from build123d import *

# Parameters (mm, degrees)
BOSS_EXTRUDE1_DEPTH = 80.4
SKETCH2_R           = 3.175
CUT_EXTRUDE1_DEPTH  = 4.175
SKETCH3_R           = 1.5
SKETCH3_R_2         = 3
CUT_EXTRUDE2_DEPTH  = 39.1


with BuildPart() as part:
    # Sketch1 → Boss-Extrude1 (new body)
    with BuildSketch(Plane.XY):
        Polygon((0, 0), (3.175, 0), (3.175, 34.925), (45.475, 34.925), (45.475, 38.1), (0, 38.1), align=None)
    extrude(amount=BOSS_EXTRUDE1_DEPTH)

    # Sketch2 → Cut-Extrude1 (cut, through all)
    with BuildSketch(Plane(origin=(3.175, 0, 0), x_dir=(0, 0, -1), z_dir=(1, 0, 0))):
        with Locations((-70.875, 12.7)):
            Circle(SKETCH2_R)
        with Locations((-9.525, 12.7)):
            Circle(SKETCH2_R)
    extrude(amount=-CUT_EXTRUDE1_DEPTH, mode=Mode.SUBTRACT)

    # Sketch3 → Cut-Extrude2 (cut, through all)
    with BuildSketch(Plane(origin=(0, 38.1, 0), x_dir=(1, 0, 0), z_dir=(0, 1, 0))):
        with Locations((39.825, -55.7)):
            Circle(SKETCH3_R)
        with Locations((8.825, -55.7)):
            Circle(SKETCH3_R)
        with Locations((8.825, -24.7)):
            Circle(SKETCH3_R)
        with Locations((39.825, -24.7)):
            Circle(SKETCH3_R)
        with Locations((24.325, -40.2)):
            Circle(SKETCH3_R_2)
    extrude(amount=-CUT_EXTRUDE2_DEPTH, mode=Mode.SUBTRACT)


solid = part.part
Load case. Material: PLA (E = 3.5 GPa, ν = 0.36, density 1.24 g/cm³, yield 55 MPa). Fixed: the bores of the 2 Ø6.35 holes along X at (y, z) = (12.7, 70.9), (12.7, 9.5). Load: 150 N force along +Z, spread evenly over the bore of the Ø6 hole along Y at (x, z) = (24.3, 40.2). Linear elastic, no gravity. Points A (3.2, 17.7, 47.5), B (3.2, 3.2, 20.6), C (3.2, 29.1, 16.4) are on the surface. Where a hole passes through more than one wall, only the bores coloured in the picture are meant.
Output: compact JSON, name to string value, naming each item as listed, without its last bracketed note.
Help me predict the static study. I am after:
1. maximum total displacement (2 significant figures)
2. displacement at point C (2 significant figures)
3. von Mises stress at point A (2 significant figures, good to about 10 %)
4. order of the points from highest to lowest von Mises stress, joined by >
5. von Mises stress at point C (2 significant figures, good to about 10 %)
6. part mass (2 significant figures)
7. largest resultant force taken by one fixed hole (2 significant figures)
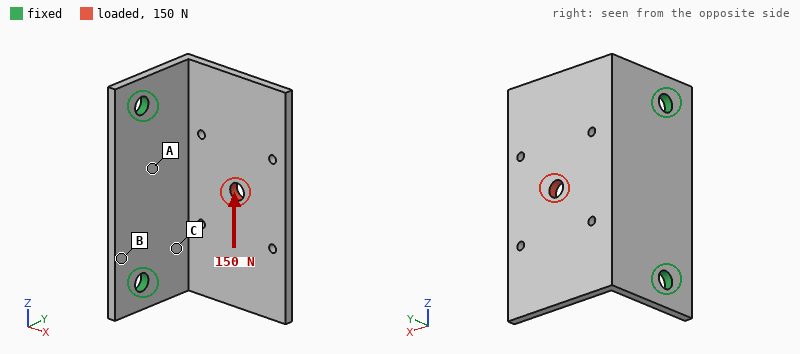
{"maximum total displacement": "1.0 mm", "displacement at point C": "0.20 mm", "von Mises stress at point A": "4.0 MPa", "order of the points from highest to lowest von Mises stress, joined by >": "C > A > B", "von Mises stress at point C": "7.6 MPa", "part mass": "25 g", "largest resultant force taken by one fixed hole": "110 N"}
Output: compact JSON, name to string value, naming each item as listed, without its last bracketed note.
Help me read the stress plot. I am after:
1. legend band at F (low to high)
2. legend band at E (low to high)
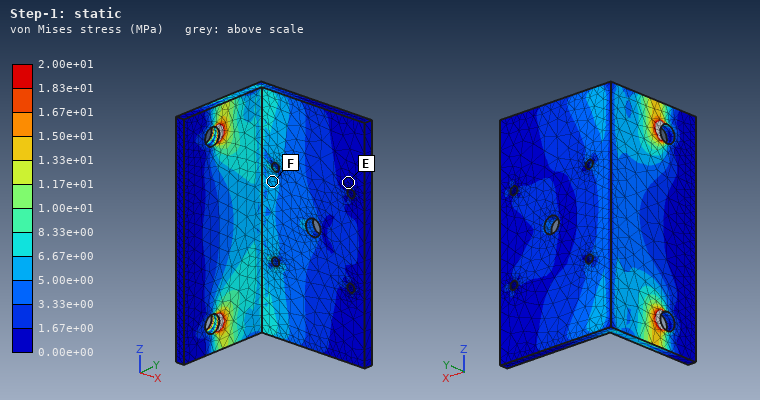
{"legend band at F": "5.00e+00 to 6.67e+00 MPa", "legend band at E": "0.00e+00 to 1.67e+00 MPa"}
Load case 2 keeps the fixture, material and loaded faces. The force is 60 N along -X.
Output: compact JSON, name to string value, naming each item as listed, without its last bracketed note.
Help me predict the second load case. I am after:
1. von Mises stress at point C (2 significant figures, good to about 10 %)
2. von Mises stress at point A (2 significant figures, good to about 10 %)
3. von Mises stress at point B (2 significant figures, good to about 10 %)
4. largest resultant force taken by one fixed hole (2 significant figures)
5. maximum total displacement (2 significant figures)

{"von Mises stress at point C": "3.5 MPa", "von Mises stress at point A": "3.0 MPa", "von Mises stress at point B": "2.6 MPa", "largest resultant force taken by one fixed hole": "30 N", "maximum total displacement": "1.1 mm"}
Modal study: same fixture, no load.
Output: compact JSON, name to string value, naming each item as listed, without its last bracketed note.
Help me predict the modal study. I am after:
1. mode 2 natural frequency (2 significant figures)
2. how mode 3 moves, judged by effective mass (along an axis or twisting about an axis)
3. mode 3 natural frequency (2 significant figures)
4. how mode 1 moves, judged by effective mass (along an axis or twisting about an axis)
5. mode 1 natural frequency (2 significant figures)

{"mode 2 natural frequency": "480 Hz", "how mode 3 moves, judged by effective mass": "along X", "mode 3 natural frequency": "740 Hz", "how mode 1 moves, judged by effective mass": "along Y", "mode 1 natural frequency": "240 Hz"}
